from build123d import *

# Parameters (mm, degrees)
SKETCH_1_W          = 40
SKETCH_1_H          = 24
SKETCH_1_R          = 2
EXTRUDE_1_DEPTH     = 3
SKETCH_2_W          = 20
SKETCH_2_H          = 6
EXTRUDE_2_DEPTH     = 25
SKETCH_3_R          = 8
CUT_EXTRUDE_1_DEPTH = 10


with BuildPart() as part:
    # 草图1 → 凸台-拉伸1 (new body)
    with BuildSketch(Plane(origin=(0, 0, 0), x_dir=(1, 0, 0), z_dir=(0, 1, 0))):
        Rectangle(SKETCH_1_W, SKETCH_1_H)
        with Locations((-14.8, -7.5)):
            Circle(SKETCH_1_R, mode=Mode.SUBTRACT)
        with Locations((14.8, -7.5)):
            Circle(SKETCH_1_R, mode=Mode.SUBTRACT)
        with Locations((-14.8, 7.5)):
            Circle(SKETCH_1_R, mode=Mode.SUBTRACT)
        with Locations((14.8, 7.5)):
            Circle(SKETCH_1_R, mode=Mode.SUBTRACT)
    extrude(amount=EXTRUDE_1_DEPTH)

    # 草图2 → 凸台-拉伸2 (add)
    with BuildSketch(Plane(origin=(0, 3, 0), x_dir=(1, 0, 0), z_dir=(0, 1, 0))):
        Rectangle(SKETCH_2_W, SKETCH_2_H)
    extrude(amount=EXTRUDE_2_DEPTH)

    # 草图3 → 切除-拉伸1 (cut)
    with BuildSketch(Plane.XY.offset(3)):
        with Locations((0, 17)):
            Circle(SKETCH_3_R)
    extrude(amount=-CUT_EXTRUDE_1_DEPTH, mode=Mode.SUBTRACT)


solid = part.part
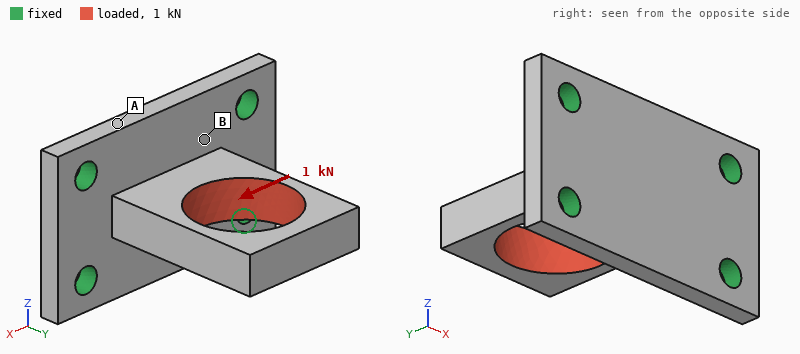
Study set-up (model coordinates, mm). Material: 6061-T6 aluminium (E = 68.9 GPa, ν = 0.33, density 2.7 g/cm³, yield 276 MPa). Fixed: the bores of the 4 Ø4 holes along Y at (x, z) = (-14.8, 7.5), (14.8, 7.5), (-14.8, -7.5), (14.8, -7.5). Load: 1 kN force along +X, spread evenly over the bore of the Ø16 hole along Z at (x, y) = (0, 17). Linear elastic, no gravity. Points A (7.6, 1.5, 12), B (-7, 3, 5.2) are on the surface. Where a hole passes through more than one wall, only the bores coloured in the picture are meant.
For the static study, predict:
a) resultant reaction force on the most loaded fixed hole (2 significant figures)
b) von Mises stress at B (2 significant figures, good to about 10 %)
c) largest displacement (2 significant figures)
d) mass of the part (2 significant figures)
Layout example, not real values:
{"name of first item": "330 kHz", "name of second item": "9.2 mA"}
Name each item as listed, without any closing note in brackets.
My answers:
{"resultant reaction force on the most loaded fixed hole": "430 N", "von Mises stress at B": "33 MPa", "largest displacement": "0.12 mm", "mass of the part": "12 g"}
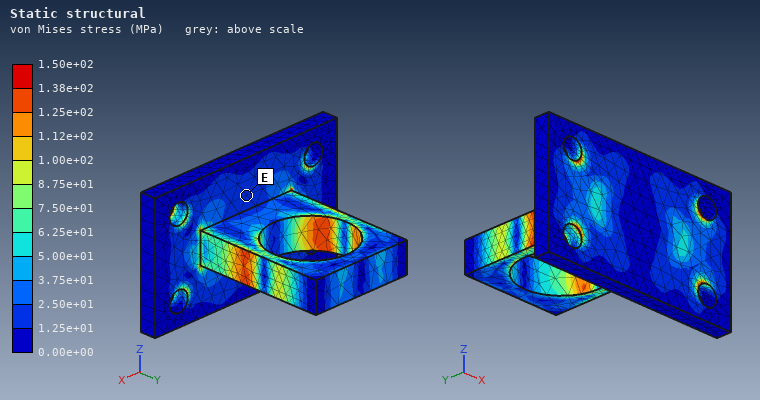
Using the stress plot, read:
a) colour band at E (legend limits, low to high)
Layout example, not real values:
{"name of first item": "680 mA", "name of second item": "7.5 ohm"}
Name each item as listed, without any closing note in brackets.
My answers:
{"colour band at E": "1.25e+01 to 2.50e+01 MPa"}
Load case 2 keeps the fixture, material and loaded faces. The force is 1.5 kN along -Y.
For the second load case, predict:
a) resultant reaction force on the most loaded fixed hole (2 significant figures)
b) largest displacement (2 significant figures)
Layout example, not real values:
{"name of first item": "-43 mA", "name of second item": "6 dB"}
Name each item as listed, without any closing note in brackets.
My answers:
{"resultant reaction force on the most loaded fixed hole": "390 N", "largest displacement": "36 µm"}
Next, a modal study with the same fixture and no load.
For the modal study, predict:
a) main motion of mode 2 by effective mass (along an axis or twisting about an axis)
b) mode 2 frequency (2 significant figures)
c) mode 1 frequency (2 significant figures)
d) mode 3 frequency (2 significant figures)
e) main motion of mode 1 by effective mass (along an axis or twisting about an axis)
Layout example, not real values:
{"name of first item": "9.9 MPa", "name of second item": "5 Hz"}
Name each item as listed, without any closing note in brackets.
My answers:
{"main motion of mode 2 by effective mass": "along X", "mode 2 frequency": "8100 Hz", "mode 1 frequency": "5000 Hz", "mode 3 frequency": "12 kHz", "main motion of mode 1 by effective mass": "along Z"}
